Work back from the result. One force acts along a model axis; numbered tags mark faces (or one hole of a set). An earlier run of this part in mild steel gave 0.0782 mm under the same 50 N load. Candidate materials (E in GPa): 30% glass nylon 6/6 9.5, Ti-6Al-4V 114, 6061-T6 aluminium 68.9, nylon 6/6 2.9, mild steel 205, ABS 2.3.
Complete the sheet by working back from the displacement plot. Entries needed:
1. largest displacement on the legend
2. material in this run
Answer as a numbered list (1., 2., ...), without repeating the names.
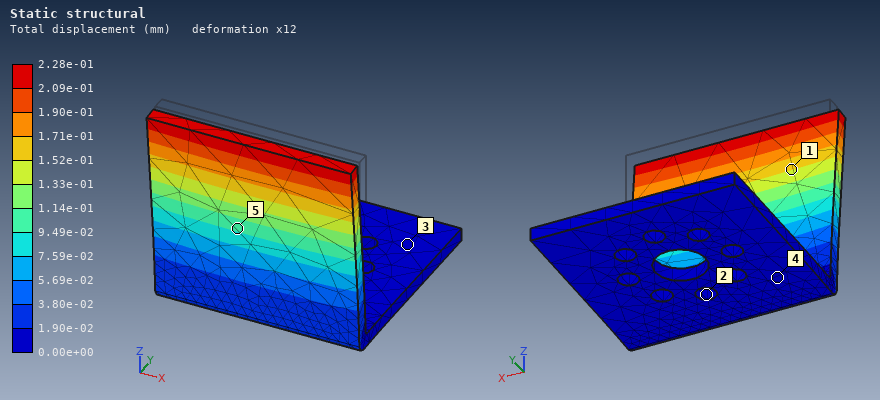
1. 2.28e-01 mm
2. 6061-T6 aluminium
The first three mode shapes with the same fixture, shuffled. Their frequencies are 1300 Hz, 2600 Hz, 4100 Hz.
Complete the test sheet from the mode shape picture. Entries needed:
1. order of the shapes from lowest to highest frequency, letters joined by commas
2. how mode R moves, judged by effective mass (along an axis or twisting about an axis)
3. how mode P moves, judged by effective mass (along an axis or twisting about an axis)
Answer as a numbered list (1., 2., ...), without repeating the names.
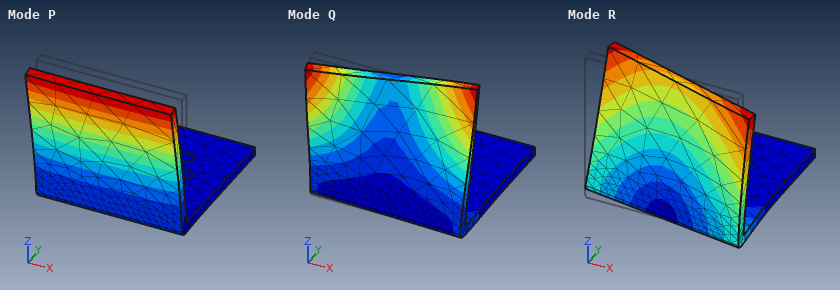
1. P, R, Q
2. along X
3. along Y
